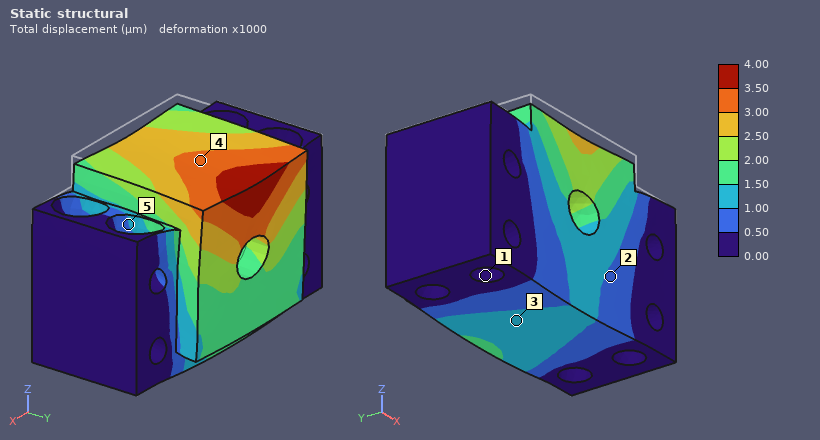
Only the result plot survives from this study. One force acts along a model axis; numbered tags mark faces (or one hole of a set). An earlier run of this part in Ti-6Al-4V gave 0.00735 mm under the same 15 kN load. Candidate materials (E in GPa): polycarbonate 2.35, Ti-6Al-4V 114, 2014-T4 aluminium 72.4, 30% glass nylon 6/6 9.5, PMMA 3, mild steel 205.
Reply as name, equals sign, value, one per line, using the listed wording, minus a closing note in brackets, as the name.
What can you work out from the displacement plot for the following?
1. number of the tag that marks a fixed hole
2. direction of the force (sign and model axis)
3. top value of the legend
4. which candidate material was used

number of the tag that marks a fixed hole = 1
direction of the force = -Z
top value of the legend = 4.00 µm
which candidate material was used = mild steel
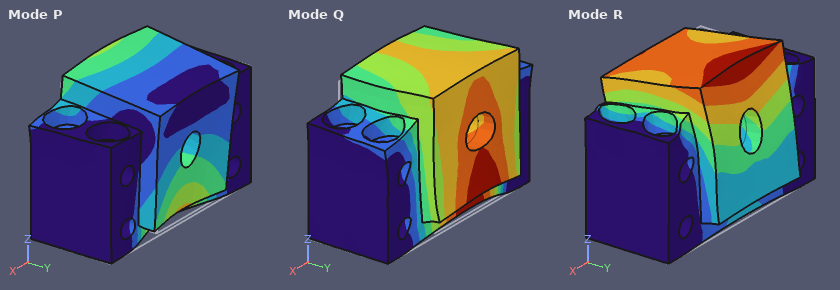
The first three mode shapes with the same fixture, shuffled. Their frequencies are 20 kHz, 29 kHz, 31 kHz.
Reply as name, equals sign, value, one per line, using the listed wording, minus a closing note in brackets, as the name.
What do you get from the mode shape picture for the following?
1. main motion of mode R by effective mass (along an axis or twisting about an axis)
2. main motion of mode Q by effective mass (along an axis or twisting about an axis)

main motion of mode R by effective mass = along Y
main motion of mode Q by effective mass = along Z
